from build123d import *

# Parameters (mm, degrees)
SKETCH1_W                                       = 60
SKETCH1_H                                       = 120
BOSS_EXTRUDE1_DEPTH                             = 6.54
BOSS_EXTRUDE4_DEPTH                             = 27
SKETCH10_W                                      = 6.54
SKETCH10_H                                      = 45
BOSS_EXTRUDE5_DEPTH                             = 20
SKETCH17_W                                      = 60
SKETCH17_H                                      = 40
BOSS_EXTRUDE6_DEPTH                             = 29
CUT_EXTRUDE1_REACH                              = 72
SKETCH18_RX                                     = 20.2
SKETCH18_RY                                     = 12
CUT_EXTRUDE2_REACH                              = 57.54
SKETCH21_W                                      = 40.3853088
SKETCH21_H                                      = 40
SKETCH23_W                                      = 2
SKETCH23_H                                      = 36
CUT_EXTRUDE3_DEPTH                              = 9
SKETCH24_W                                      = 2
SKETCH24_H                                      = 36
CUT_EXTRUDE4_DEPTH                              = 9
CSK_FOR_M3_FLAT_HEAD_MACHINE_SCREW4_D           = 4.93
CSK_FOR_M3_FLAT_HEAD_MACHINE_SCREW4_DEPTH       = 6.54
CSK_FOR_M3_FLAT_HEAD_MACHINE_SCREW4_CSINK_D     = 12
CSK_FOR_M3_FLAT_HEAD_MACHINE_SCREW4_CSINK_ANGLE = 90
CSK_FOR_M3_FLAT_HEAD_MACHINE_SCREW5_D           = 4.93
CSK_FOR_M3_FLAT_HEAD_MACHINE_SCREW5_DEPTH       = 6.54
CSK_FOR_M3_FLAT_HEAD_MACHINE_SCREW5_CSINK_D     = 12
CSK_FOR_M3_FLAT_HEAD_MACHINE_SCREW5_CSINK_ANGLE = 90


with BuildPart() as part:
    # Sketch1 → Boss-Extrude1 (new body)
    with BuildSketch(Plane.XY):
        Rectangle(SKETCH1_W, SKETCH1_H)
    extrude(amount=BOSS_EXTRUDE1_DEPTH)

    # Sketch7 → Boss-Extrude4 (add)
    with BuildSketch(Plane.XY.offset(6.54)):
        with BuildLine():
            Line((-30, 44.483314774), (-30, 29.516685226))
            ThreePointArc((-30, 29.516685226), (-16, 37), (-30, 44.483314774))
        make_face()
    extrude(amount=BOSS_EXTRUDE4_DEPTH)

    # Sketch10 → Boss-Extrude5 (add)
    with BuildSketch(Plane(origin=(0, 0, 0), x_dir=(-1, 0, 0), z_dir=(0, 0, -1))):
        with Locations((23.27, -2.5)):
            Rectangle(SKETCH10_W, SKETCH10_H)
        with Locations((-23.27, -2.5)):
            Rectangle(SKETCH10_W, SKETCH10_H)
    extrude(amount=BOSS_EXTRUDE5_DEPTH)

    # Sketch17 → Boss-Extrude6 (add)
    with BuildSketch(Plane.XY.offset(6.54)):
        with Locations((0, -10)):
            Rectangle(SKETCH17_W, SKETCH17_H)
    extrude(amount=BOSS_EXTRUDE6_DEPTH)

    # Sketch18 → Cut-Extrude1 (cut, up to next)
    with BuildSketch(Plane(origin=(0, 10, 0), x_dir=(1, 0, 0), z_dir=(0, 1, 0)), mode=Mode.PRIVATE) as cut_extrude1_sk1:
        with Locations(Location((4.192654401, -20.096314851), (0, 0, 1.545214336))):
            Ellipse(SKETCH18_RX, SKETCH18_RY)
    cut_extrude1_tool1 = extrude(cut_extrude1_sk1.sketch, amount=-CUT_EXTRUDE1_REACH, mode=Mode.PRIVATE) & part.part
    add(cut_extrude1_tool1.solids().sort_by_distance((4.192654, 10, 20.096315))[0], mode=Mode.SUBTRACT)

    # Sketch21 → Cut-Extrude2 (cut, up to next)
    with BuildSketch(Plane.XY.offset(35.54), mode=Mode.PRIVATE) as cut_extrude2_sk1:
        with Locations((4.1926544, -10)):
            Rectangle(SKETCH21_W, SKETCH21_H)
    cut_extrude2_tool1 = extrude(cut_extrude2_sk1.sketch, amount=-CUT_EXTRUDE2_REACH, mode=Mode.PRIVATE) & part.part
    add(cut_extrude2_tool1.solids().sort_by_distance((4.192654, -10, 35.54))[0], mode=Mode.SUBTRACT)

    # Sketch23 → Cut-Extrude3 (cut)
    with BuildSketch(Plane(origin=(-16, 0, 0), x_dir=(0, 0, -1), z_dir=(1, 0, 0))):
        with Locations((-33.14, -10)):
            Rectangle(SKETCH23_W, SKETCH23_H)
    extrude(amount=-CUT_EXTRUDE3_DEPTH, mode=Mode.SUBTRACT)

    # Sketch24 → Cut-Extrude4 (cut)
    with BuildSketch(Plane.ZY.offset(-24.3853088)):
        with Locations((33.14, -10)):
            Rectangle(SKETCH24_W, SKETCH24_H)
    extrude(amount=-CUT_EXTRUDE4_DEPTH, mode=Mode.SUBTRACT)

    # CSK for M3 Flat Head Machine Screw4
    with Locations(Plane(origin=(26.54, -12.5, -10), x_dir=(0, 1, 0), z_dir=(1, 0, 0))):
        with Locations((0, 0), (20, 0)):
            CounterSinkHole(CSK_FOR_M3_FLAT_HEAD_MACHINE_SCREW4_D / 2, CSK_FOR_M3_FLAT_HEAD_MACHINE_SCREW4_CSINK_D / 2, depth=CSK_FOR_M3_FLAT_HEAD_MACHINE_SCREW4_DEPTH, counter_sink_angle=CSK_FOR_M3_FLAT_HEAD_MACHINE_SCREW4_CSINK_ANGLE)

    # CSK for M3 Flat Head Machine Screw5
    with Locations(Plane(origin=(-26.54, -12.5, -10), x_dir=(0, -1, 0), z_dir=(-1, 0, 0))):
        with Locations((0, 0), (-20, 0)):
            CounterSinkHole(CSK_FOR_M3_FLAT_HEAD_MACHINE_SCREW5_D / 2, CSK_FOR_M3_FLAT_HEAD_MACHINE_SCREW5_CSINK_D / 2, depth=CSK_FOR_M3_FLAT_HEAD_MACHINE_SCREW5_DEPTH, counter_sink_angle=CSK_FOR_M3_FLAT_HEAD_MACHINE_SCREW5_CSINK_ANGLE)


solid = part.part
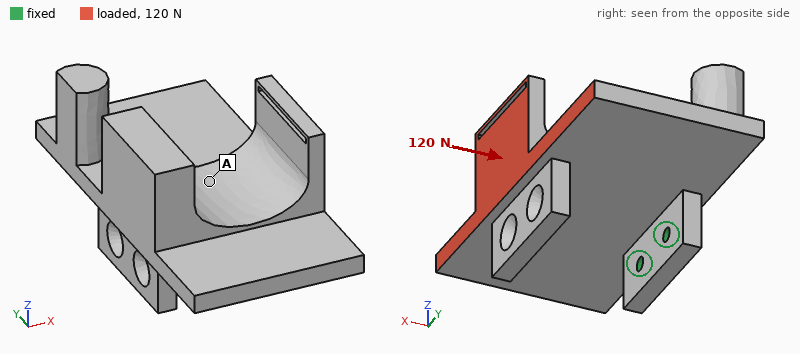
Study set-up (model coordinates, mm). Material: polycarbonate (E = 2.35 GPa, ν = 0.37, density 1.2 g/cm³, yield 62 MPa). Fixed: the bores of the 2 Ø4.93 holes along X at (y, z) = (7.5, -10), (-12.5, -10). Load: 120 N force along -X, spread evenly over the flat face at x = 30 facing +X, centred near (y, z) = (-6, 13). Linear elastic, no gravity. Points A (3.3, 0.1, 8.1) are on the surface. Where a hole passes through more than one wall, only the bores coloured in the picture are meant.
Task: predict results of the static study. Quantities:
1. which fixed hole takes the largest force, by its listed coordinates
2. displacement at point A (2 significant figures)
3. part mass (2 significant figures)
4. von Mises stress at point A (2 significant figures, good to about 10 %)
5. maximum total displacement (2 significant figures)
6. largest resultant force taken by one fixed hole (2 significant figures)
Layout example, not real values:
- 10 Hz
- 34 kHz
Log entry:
- (-12.5, -10)
- 0.60 mm
- 110 g
- 1.8 MPa
- 1.6 mm
- 77 N
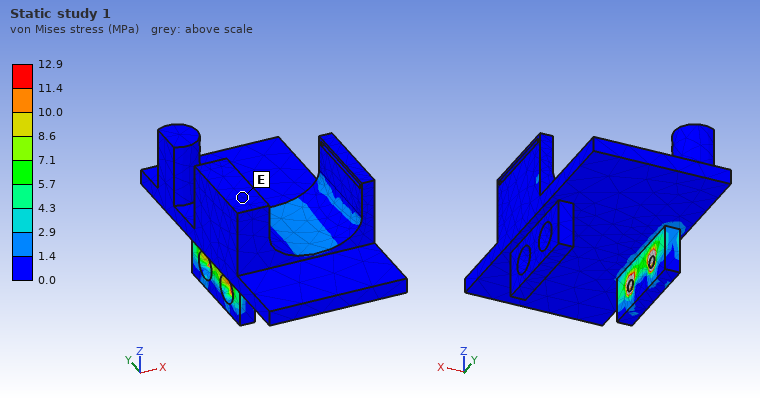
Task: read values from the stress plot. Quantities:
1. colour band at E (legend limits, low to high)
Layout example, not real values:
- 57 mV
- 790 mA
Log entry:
- 0.0 to 1.4 MPa
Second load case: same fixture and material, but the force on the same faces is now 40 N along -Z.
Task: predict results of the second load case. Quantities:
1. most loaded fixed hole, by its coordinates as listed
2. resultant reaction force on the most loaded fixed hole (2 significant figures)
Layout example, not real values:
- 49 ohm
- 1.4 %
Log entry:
- (-12.5, -10)
- 31 N
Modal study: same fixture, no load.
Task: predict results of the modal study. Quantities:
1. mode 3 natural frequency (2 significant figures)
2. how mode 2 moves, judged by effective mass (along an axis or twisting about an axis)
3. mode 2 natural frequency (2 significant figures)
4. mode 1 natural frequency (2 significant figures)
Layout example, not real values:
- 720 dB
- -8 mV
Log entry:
- 440 Hz
- along Y
- 310 Hz
- 160 Hz
